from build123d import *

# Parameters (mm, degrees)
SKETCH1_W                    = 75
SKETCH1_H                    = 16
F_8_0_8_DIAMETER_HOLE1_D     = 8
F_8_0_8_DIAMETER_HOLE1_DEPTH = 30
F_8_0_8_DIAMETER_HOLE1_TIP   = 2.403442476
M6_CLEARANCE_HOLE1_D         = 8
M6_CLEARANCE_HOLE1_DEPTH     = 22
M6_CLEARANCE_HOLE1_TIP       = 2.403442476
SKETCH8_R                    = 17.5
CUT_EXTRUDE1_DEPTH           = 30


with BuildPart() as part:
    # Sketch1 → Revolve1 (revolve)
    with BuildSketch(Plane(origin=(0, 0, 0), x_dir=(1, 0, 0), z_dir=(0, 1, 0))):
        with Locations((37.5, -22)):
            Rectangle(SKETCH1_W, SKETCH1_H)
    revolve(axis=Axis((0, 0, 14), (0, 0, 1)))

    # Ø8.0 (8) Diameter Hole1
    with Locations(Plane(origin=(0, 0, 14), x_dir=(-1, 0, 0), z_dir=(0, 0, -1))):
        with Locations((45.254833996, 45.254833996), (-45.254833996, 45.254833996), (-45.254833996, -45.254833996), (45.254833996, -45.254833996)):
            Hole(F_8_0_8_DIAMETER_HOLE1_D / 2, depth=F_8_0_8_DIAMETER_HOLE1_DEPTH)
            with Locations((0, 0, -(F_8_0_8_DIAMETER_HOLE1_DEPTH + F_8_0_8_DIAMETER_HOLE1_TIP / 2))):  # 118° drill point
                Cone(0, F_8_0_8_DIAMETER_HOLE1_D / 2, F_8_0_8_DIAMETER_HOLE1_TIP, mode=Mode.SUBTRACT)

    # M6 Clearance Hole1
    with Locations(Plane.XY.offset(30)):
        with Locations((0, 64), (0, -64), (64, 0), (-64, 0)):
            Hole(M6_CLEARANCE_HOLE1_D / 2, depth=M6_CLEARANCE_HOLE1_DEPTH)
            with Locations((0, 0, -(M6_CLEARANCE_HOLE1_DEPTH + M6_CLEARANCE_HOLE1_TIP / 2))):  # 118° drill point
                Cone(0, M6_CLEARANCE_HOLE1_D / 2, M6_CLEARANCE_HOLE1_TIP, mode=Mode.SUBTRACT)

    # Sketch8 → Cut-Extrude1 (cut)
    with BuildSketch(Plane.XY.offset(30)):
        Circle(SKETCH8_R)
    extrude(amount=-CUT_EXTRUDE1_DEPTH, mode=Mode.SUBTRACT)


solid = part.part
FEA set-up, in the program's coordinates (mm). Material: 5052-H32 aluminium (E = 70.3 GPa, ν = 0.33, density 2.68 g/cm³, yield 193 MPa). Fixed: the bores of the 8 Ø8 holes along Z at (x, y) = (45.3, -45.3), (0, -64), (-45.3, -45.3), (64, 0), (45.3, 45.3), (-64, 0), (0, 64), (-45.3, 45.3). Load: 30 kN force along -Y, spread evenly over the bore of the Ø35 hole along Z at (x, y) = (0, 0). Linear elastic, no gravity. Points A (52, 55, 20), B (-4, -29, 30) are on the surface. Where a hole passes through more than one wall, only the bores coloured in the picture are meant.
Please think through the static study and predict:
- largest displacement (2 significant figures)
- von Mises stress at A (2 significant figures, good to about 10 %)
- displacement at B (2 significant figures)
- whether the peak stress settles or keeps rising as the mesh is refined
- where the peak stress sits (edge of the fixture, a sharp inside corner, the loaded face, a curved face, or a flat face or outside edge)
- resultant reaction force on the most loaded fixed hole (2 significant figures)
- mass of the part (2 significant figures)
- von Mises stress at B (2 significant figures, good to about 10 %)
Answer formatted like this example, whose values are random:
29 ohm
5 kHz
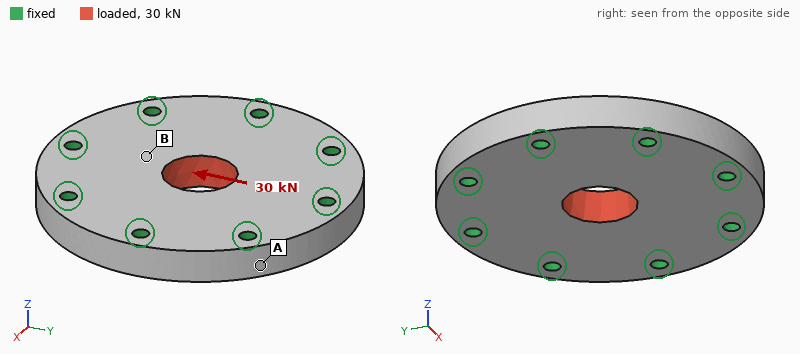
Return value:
10 µm
5.3 MPa
7.2 µm
keeps rising
edge of the fixture
6.2 kN
700 g
15 MPa
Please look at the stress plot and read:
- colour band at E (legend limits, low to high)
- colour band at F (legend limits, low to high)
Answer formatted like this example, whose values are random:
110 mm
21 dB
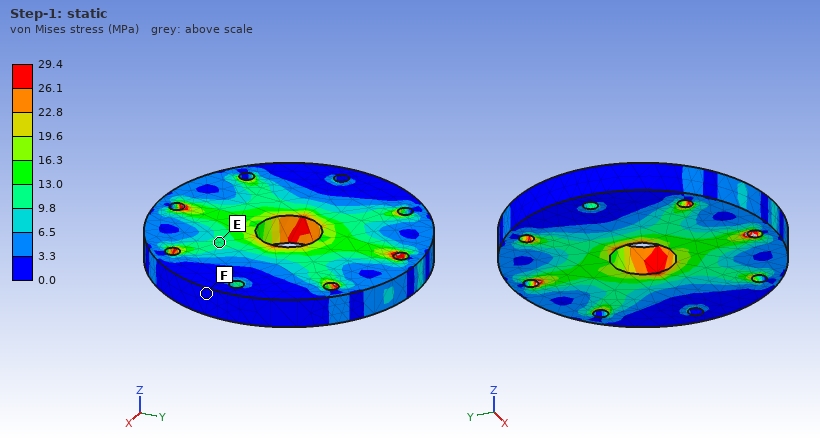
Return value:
9.8 to 13.0 MPa
0.0 to 3.3 MPa
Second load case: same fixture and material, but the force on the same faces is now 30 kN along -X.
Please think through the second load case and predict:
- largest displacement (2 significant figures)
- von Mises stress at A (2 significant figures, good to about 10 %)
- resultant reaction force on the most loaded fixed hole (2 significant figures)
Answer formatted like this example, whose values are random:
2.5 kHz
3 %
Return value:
10 µm
4.8 MPa
6.2 kN
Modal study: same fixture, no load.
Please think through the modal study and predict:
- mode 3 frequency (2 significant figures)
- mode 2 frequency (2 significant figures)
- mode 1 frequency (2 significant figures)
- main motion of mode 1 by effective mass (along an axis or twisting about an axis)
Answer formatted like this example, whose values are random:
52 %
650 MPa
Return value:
13 kHz
13 kHz
8000 Hz
along Z
